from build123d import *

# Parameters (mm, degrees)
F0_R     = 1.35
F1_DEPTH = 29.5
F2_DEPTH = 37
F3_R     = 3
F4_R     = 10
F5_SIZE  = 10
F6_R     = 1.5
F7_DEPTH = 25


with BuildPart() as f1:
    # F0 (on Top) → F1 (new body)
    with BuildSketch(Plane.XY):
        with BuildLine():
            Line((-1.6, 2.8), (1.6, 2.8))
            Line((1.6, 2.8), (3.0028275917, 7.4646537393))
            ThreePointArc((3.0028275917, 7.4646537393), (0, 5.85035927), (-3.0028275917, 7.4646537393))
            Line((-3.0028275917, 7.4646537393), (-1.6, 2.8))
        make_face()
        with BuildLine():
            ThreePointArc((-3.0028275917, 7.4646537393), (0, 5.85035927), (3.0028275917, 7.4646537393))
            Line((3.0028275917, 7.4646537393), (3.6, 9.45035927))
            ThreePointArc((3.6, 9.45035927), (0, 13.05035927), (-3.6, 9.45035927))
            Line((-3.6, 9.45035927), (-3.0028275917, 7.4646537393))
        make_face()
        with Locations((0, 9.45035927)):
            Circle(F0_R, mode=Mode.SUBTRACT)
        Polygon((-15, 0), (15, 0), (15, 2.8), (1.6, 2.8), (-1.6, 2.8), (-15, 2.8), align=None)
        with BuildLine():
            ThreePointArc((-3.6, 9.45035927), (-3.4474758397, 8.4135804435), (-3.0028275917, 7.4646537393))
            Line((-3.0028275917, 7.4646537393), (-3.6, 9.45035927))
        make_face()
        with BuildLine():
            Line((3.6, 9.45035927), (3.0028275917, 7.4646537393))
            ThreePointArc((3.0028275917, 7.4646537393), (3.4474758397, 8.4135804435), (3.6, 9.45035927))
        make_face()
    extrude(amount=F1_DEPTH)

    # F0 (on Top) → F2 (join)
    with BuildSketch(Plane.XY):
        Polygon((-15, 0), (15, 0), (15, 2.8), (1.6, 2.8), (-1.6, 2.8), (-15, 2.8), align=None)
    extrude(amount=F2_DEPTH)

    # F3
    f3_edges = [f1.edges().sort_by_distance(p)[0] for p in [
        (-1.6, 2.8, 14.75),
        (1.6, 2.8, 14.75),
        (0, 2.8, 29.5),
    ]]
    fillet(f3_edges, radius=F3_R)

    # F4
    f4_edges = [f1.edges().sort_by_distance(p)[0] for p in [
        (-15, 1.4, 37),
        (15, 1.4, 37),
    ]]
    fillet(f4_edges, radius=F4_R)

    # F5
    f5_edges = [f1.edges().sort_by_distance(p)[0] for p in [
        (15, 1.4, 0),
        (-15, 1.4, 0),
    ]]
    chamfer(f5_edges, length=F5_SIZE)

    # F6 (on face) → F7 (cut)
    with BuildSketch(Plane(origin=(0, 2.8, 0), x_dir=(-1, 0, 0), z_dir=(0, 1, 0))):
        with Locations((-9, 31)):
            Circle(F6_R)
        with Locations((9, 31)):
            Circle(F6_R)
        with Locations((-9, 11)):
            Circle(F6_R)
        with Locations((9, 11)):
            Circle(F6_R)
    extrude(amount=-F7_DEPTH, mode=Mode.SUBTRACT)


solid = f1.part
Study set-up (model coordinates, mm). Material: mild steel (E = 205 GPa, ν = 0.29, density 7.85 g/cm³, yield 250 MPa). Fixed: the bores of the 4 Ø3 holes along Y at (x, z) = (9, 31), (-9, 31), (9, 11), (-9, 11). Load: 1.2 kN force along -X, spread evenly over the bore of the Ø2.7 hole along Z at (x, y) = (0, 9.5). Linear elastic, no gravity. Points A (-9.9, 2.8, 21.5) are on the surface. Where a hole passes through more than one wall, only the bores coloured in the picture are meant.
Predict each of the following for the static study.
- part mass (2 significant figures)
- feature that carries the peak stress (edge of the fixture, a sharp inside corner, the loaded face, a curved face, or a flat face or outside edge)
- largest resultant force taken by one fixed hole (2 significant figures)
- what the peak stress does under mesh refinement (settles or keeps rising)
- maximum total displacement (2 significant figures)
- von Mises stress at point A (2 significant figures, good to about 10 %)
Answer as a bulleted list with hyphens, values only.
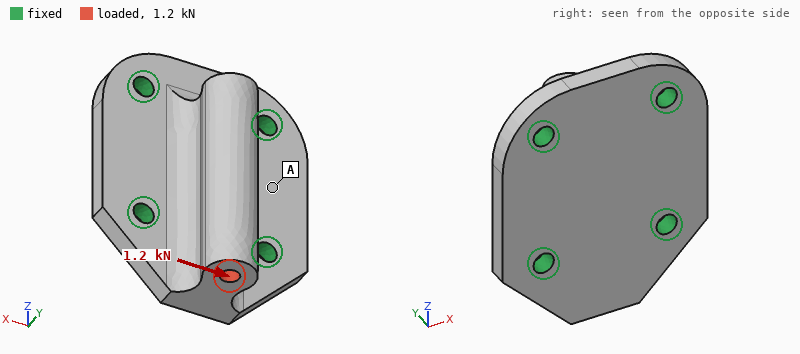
- 34 g
- edge of the fixture
- 620 N
- keeps rising
- 8.4 µm
- 11 MPa
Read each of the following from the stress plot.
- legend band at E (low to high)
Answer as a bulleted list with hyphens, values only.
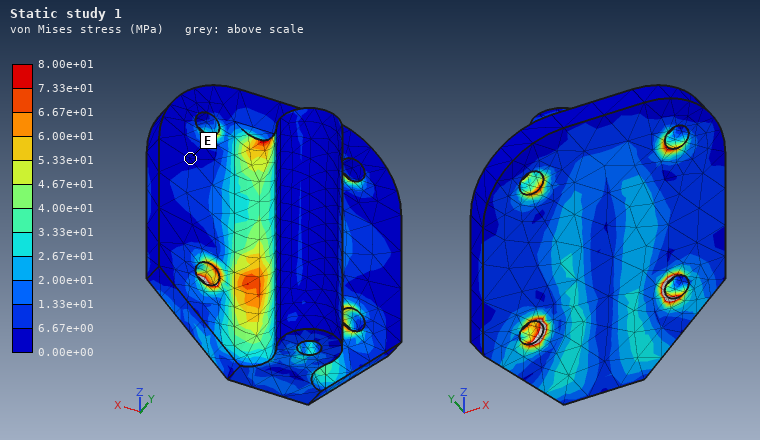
- 0.00e+00 to 6.67e+00 MPa
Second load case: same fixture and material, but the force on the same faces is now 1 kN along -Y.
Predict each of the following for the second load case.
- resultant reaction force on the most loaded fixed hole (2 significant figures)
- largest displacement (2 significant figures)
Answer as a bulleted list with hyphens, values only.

- 420 N
- 4.1 µm
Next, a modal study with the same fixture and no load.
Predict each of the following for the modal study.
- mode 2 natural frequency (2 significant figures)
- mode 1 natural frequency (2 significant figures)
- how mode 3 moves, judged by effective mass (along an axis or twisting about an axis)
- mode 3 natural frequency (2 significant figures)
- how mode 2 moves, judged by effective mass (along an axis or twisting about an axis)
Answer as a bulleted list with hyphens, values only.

- 23 kHz
- 19 kHz
- along Y
- 26 kHz
- along X
